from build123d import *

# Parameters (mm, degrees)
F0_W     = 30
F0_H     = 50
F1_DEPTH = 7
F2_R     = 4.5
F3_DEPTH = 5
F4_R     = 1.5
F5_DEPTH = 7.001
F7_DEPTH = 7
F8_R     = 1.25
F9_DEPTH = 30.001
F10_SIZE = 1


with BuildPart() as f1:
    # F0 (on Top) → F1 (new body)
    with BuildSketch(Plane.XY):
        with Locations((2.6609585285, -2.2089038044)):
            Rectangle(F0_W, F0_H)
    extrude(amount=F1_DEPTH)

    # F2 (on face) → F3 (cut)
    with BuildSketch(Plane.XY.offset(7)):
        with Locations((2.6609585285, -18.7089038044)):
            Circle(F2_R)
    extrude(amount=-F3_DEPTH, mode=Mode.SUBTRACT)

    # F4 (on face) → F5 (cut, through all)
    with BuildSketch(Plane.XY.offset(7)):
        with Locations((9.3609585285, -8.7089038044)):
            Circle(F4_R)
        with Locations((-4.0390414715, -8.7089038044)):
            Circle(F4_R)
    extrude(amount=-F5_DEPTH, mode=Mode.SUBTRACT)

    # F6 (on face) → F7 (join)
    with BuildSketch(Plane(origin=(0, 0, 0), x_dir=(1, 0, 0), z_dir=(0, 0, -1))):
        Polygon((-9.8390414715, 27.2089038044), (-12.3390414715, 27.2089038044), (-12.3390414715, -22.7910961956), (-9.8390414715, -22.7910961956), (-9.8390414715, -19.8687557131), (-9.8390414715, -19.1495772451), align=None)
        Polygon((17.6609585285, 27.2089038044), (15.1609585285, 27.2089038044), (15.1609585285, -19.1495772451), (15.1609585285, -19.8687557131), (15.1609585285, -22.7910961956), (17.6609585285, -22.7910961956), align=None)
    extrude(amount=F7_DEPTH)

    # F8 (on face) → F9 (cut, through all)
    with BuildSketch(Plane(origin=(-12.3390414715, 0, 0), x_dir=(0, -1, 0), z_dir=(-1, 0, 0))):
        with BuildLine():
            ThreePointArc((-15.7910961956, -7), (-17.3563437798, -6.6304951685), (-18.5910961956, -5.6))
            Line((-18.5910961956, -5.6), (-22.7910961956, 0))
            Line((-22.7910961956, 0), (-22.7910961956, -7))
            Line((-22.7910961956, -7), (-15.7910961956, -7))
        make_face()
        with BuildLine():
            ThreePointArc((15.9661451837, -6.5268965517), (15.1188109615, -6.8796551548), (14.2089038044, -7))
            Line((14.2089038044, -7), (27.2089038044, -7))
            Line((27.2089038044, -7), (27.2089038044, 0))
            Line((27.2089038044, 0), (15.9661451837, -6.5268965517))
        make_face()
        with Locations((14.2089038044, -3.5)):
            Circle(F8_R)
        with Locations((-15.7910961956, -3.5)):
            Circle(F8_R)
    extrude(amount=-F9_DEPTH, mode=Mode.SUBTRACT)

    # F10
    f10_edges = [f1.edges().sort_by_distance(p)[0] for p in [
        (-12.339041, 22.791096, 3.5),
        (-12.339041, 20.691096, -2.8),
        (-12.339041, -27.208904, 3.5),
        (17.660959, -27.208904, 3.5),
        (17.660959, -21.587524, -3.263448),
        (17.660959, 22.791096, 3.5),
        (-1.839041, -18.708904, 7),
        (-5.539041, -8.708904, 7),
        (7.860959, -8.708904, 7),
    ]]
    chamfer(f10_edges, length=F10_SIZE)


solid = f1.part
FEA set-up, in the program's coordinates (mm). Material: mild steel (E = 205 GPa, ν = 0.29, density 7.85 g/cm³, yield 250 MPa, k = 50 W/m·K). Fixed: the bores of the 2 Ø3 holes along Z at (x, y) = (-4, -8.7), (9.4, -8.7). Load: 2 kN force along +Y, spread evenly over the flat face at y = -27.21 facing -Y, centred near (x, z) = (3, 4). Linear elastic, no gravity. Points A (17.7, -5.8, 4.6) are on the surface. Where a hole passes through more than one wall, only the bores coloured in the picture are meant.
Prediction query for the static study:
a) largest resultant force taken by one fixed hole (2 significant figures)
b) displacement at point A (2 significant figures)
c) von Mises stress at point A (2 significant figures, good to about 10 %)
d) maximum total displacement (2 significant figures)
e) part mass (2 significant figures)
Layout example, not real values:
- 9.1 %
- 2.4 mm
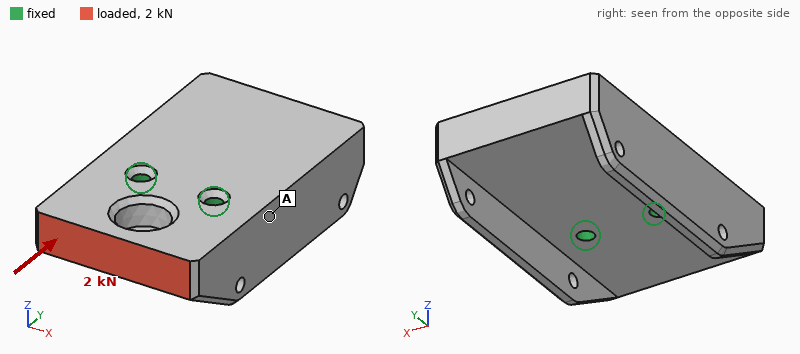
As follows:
- 1.0 kN
- 0.40 µm
- 6.6 MPa
- 2.6 µm
- 89 g
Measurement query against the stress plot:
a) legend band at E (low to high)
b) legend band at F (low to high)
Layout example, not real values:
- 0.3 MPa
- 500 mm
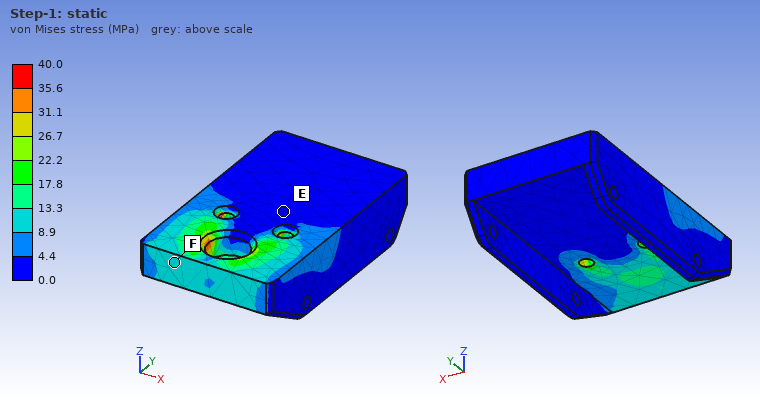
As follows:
- 0.0 to 4.4 MPa
- 8.9 to 13.3 MPa
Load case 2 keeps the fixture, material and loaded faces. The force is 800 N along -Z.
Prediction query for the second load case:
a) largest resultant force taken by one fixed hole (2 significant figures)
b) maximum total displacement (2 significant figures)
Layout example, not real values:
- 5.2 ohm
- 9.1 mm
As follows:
- 400 N
- 14 µm
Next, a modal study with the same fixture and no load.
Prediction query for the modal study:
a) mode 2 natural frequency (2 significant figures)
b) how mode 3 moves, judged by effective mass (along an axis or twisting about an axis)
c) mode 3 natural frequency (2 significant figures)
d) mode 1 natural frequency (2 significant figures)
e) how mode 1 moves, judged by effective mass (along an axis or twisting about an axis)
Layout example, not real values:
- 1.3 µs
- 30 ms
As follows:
- 11 kHz
- along X
- 12 kHz
- 5500 Hz
- along Z
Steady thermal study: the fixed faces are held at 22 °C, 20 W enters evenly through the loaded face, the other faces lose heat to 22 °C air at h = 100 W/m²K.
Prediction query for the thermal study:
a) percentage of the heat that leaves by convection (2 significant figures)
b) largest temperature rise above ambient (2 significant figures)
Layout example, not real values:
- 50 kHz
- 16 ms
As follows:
- 20 %
- 40 K
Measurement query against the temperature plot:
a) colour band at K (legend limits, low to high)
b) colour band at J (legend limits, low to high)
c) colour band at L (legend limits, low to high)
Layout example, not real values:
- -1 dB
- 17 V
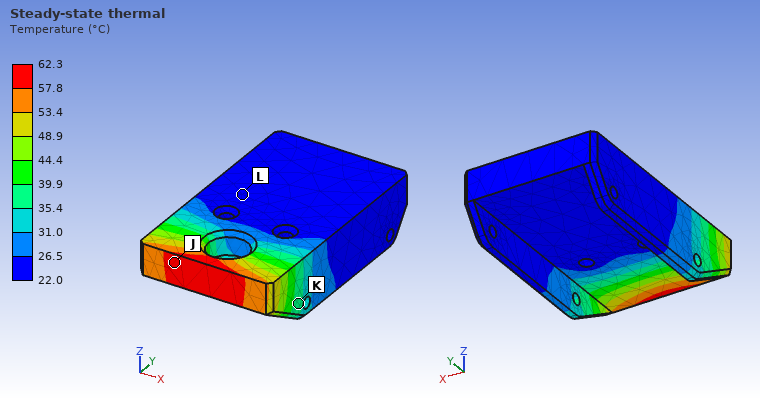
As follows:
- 35.4 to 39.9 °C
- 57.8 to 62.3 °C
- 22.0 to 26.5 °C
